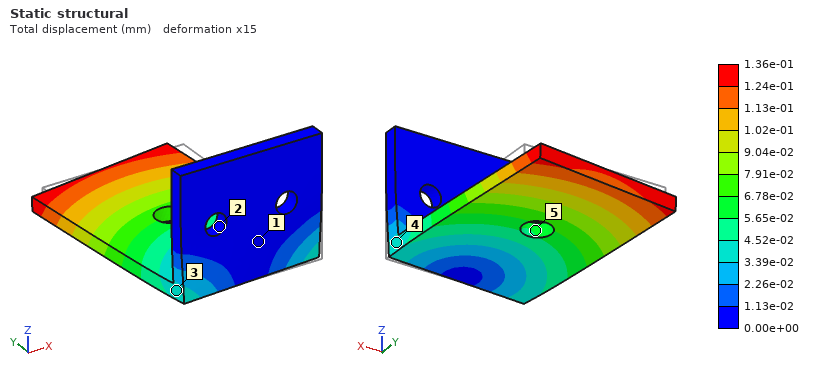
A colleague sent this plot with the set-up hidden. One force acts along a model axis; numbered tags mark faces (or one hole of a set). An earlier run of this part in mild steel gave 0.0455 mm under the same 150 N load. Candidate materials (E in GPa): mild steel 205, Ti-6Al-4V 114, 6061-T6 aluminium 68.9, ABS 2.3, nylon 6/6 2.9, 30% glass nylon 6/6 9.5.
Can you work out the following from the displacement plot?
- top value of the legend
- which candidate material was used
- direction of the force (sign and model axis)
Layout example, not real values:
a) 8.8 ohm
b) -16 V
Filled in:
a) 1.36e-01 mm
b) 6061-T6 aluminium
c) -X
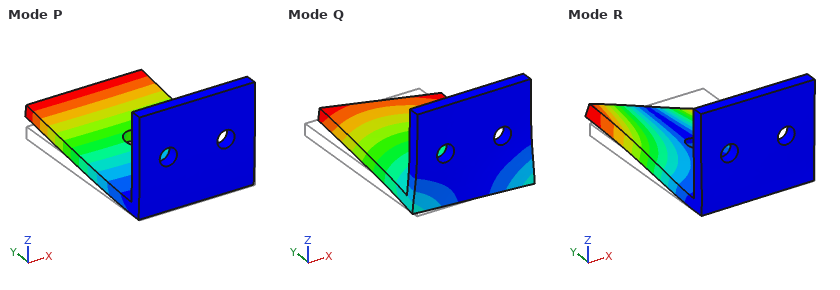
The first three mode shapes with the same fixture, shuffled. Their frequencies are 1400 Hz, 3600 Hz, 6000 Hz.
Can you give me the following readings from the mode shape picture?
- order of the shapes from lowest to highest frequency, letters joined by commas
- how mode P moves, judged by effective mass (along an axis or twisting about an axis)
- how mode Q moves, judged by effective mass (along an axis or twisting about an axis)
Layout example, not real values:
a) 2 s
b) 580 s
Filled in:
a) P, Q, R
b) along Z
c) along X
